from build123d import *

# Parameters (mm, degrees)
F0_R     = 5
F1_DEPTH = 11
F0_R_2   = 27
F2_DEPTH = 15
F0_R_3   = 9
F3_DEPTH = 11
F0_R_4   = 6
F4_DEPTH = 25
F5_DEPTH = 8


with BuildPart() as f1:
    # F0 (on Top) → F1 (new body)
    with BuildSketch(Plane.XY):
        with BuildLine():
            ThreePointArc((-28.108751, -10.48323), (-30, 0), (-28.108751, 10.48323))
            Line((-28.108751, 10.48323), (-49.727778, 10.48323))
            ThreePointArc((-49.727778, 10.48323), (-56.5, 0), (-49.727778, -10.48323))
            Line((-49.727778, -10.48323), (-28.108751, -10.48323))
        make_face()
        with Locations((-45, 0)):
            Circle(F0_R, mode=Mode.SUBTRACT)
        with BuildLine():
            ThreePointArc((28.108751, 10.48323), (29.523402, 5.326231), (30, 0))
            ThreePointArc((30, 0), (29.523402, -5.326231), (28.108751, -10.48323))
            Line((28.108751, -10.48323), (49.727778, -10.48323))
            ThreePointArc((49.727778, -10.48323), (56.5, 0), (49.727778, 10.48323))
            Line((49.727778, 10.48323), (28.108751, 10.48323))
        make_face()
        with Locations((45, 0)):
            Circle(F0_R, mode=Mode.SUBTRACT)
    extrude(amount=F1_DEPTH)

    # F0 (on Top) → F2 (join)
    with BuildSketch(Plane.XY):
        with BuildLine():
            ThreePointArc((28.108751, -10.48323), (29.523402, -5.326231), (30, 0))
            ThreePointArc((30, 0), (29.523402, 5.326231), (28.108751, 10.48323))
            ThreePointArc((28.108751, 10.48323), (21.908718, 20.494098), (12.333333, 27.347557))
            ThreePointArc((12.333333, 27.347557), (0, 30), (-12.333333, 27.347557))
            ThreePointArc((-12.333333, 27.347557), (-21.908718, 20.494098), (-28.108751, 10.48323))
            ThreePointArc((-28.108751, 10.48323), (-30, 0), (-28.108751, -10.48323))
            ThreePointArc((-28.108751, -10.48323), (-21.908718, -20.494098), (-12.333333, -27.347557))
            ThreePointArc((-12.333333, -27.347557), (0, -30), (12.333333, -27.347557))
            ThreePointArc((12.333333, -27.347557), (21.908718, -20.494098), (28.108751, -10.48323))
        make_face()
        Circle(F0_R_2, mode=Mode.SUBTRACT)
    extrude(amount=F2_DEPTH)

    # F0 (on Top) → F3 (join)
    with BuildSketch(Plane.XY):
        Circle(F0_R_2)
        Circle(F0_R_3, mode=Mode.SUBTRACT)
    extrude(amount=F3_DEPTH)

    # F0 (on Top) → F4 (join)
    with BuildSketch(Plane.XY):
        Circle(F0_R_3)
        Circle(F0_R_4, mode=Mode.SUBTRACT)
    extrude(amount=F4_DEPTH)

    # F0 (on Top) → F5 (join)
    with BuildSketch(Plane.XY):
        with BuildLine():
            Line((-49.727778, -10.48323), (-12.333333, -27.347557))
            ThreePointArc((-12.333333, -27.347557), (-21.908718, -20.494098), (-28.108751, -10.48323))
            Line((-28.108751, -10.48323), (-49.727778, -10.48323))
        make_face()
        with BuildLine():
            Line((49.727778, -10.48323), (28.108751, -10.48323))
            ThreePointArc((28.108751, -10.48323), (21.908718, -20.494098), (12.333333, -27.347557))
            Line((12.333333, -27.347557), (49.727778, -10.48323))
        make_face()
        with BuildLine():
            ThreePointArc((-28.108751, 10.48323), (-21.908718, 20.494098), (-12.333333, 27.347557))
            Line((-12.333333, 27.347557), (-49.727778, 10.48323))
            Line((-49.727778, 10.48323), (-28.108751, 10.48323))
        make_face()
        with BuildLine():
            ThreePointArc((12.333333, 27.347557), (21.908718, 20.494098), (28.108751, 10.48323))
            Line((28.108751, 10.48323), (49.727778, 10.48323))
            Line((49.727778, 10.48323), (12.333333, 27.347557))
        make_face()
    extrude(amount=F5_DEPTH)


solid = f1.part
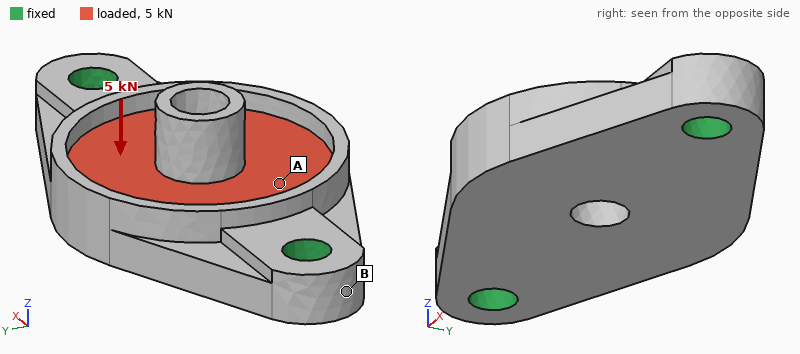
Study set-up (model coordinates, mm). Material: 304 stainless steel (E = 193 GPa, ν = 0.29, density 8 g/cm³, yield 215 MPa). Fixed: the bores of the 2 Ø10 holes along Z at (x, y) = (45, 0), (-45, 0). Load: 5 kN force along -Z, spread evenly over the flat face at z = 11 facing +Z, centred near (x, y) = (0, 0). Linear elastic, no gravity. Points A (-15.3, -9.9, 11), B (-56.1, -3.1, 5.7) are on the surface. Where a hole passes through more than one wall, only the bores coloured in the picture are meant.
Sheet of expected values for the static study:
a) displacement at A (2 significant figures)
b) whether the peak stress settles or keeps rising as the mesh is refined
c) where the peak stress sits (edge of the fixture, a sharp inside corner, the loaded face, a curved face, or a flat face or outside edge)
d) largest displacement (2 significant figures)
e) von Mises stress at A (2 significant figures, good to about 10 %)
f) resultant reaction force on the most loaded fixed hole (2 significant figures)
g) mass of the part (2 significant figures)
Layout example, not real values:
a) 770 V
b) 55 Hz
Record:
a) 15 µm
b) keeps rising
c) edge of the fixture
d) 22 µm
e) 24 MPa
f) 2.5 kN
g) 390 g
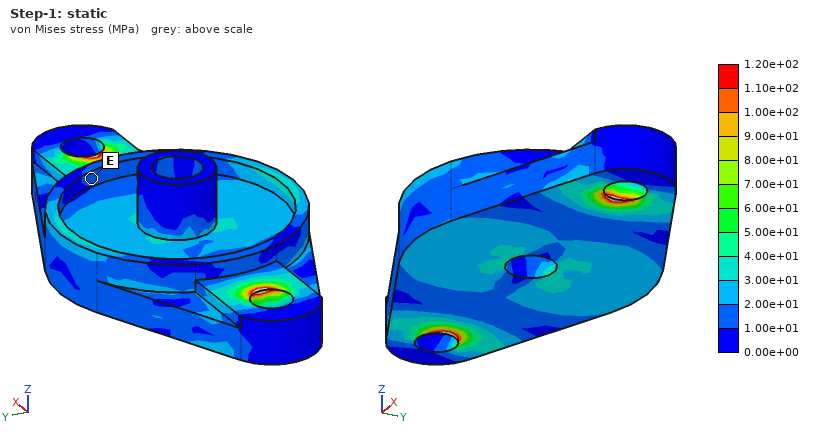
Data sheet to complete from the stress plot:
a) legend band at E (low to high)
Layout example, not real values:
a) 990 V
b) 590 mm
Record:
a) 1.00e+01 to 2.00e+01 MPa
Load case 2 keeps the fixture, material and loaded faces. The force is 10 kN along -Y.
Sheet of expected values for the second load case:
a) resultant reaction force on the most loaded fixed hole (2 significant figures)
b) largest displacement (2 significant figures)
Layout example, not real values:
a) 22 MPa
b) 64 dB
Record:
a) 5.0 kN
b) 30 µm
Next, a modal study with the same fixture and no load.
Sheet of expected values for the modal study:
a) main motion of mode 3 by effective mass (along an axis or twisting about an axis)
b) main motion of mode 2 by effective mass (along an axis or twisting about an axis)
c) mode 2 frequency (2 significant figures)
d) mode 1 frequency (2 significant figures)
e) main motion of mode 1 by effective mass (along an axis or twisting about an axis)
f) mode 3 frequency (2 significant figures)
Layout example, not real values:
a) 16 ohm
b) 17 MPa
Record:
a) along Y
b) along Z
c) 5200 Hz
d) 5000 Hz
e) twisting about X
f) 11 kHz
